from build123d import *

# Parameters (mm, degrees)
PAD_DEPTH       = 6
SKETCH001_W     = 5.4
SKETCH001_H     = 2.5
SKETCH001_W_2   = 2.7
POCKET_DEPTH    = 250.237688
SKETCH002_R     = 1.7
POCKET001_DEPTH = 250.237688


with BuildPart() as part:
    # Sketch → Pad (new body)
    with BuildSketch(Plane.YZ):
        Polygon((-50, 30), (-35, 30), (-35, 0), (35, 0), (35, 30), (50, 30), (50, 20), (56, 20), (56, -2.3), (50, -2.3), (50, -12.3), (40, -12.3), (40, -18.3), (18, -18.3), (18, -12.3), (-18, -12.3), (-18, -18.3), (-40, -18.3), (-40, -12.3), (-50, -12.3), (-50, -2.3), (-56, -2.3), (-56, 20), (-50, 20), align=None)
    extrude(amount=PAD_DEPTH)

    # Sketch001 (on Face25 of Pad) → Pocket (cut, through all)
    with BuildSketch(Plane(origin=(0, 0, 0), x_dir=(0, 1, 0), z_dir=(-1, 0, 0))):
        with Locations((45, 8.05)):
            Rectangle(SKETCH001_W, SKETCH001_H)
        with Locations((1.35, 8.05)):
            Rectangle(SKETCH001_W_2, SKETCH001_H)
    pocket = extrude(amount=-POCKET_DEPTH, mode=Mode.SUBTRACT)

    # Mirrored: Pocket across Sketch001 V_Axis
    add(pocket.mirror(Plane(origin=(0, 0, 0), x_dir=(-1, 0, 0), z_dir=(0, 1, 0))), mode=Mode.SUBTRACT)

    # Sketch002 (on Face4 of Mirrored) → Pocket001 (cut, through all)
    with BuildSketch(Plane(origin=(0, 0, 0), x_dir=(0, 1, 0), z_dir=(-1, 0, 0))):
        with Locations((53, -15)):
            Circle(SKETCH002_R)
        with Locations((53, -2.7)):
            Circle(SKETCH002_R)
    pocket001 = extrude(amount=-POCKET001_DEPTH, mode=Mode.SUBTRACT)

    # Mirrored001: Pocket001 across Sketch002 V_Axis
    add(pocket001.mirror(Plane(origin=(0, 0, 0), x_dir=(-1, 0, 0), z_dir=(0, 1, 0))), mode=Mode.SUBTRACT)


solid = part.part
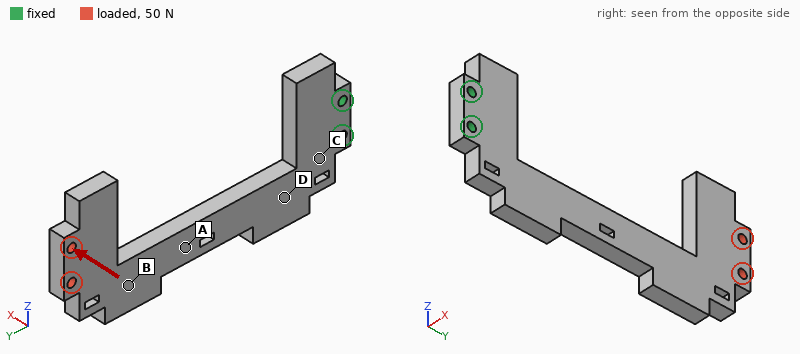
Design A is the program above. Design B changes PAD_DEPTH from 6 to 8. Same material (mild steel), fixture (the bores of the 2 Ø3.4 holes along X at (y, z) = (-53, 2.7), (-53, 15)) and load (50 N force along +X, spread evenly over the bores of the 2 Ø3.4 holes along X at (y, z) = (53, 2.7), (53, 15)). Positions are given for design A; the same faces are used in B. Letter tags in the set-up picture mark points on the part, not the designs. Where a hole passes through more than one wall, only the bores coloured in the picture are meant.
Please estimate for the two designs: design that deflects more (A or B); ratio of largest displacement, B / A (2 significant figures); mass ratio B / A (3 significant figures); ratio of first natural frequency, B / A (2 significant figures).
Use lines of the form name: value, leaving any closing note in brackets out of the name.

design that deflects more: A
ratio of largest displacement, B / A: 0.44
mass ratio B / A: 1.33
ratio of first natural frequency, B / A: 1.3
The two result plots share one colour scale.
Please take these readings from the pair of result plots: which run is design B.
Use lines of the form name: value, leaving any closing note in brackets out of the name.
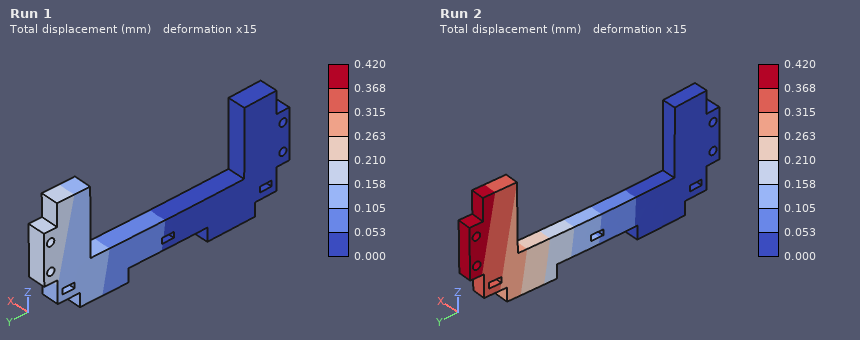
which run is design B: Run 1
